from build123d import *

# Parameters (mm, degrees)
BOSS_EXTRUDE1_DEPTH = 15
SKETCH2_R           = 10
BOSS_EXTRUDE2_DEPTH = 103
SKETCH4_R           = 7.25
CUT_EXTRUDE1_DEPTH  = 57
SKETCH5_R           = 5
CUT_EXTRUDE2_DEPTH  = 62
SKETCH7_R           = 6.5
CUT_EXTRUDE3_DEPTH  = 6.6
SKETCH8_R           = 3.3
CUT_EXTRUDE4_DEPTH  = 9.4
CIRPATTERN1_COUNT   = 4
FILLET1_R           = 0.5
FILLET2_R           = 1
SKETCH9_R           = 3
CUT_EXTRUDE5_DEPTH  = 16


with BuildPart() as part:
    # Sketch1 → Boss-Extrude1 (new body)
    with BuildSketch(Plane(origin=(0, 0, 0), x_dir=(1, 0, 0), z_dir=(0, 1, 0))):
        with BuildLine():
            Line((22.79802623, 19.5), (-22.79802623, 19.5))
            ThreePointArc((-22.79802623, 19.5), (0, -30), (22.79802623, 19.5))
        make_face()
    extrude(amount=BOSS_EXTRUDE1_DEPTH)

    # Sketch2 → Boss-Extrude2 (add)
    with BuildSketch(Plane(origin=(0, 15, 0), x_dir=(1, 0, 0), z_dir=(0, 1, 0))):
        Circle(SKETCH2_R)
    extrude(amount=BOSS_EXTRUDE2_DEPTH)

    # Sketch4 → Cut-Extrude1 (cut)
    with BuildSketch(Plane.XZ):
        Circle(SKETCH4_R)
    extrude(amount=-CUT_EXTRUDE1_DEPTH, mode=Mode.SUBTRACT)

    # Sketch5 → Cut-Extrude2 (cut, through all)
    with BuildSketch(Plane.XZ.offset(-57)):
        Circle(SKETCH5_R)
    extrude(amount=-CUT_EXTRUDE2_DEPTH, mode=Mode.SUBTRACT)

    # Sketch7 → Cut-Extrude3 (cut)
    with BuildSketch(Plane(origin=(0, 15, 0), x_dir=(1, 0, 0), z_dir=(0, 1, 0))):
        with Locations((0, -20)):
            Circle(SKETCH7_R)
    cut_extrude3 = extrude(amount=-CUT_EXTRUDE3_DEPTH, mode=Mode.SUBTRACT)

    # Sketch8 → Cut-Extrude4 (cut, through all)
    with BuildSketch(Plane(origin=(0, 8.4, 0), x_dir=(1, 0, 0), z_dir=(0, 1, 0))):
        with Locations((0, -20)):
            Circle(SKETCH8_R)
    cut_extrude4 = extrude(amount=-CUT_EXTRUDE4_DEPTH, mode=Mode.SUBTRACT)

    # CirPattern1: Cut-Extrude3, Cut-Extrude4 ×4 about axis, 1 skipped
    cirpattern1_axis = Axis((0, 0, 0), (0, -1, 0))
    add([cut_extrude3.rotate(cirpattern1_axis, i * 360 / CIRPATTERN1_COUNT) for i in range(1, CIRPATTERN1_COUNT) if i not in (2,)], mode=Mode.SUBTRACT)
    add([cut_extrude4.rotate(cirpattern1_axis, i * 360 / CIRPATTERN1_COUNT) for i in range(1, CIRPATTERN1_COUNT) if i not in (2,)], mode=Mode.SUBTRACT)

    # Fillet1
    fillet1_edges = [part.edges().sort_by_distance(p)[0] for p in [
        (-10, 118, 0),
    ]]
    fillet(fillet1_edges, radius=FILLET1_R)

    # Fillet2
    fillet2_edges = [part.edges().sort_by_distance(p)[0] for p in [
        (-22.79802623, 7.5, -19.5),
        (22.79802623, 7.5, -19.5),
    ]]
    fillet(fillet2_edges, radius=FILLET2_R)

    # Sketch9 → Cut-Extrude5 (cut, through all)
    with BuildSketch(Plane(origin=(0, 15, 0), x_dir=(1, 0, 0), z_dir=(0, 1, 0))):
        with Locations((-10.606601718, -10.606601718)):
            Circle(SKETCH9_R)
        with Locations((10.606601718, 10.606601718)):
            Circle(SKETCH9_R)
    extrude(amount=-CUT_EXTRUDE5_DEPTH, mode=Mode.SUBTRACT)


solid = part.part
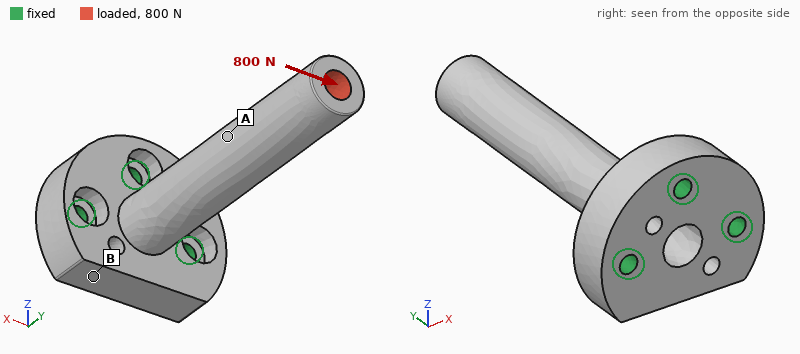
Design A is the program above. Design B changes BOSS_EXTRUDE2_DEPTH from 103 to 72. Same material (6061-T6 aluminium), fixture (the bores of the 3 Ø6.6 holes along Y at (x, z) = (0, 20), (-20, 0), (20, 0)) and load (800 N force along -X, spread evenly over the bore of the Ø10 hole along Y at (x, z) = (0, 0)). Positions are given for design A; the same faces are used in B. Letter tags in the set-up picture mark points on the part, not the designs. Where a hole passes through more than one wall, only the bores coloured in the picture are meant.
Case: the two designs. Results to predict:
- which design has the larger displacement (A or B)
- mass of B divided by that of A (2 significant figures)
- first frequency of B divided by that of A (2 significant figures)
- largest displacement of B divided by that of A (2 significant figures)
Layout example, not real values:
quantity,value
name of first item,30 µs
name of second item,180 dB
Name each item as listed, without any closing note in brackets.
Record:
quantity,value
which design has the larger displacement,A
mass of B divided by that of A,0.86
first frequency of B divided by that of A,1.9
largest displacement of B divided by that of A,0.46
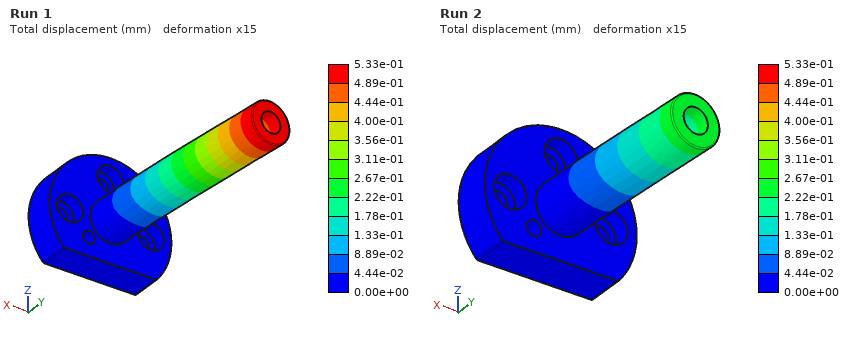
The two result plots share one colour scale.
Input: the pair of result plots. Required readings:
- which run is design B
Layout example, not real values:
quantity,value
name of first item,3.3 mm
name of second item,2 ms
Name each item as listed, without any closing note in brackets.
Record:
quantity,value
which run is design B,Run 2
